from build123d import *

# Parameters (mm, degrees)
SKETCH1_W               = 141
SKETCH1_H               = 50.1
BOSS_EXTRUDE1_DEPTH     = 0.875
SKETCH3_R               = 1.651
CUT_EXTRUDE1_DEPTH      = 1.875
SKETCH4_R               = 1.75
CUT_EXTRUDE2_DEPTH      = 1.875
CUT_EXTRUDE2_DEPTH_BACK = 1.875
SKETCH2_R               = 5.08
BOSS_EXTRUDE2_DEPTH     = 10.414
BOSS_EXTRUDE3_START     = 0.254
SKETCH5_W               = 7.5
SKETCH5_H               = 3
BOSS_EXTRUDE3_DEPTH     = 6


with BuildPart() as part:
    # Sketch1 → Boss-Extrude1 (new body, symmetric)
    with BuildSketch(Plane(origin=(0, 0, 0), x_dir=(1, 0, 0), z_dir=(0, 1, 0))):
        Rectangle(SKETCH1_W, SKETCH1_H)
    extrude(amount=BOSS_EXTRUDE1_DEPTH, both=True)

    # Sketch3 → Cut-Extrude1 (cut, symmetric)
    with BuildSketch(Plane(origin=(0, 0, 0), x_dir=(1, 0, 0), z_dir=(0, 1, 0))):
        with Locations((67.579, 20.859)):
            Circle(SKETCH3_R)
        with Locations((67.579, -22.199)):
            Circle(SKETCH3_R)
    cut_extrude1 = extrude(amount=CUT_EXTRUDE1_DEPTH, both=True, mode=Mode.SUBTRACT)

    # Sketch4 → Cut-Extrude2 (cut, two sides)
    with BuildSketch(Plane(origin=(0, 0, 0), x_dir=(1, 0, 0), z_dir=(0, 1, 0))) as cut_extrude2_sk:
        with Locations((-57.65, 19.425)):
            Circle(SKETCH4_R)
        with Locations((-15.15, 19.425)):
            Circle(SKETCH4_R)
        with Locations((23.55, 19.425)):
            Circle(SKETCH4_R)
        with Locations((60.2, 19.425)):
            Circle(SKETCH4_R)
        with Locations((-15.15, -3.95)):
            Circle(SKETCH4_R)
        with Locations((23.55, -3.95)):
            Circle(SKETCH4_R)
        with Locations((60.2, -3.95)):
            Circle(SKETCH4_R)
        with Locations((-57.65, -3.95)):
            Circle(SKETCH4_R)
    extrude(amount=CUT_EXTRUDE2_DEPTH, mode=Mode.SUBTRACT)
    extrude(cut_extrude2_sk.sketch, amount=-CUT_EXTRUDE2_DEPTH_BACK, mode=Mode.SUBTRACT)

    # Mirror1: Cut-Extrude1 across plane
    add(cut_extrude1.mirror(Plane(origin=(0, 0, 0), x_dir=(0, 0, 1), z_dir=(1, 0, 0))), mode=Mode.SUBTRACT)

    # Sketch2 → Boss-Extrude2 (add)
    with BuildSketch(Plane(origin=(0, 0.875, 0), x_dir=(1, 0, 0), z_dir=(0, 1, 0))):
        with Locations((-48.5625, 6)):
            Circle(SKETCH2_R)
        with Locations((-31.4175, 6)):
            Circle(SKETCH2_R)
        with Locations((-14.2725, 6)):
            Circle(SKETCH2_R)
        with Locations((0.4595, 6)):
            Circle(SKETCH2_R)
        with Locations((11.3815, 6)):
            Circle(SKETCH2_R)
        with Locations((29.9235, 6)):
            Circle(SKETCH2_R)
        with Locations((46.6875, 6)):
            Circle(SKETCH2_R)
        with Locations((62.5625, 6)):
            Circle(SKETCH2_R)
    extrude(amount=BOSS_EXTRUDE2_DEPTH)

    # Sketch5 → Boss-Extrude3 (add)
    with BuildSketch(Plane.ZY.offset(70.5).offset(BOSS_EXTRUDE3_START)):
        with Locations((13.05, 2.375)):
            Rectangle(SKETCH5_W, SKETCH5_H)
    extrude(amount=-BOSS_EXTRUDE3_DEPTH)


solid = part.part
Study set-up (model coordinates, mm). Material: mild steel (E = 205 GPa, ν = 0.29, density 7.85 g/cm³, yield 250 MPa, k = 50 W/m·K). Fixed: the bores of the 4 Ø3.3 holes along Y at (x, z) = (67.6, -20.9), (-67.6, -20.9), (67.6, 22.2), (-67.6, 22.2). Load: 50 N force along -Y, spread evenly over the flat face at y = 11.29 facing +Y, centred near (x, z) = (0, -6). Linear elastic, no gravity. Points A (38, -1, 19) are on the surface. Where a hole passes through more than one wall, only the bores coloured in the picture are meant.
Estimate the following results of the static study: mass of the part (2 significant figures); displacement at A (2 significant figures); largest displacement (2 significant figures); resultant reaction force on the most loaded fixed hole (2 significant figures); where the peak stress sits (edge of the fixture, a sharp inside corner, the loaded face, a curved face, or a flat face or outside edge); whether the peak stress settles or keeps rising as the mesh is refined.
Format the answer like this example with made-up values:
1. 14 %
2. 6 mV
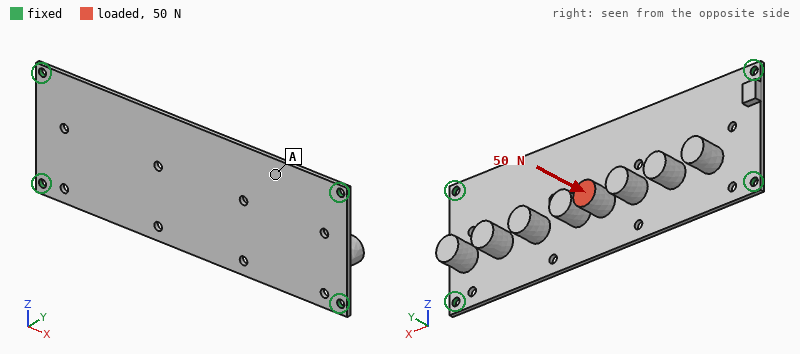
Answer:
1. 150 g
2. 0.058 mm
3. 0.15 mm
4. 19 N
5. edge of the fixture
6. keeps rising
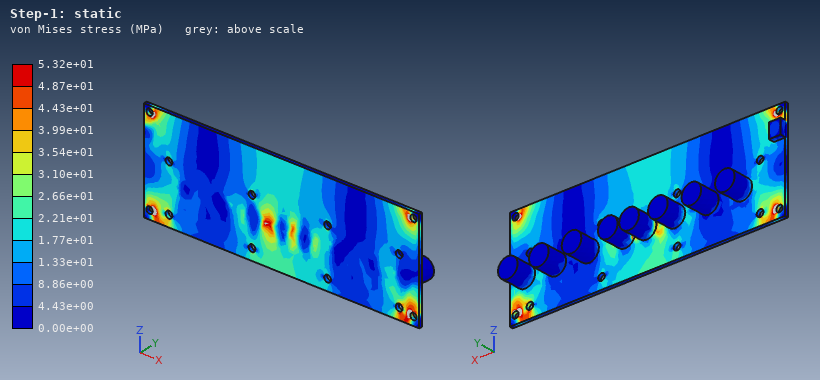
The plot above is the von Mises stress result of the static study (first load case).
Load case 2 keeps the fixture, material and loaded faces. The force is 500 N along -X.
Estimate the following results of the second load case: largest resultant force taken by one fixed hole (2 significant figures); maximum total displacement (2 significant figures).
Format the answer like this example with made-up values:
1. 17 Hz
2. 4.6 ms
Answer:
1. 150 N
2. 0.13 mm
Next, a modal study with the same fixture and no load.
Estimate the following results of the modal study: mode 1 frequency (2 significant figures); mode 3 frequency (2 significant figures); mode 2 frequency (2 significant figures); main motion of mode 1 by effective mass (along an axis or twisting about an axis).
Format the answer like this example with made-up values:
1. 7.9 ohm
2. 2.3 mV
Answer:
1. 380 Hz
2. 1100 Hz
3. 1100 Hz
4. along Y
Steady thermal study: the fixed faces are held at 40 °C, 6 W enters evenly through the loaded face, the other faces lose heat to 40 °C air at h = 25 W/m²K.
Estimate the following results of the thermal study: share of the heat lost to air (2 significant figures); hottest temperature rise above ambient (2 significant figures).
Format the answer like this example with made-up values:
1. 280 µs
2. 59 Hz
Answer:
1. 74 %
2. 45 K
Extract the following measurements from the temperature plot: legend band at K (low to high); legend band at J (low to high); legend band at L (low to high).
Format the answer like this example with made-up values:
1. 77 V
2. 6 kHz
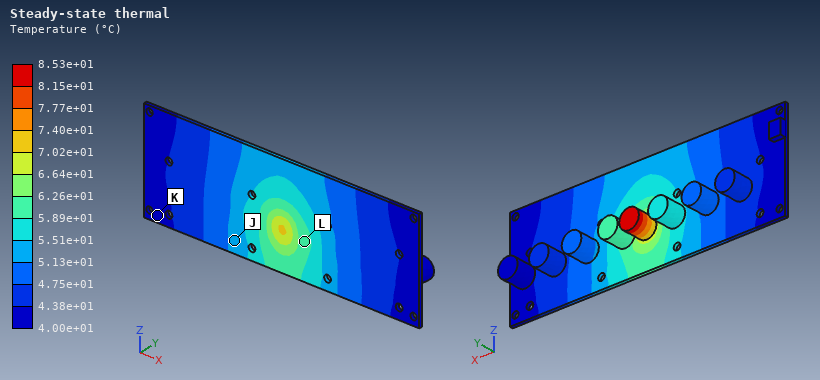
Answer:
1. 4.00e+01 to 4.38e+01 °C
2. 5.13e+01 to 5.51e+01 °C
3. 5.89e+01 to 6.26e+01 °C
